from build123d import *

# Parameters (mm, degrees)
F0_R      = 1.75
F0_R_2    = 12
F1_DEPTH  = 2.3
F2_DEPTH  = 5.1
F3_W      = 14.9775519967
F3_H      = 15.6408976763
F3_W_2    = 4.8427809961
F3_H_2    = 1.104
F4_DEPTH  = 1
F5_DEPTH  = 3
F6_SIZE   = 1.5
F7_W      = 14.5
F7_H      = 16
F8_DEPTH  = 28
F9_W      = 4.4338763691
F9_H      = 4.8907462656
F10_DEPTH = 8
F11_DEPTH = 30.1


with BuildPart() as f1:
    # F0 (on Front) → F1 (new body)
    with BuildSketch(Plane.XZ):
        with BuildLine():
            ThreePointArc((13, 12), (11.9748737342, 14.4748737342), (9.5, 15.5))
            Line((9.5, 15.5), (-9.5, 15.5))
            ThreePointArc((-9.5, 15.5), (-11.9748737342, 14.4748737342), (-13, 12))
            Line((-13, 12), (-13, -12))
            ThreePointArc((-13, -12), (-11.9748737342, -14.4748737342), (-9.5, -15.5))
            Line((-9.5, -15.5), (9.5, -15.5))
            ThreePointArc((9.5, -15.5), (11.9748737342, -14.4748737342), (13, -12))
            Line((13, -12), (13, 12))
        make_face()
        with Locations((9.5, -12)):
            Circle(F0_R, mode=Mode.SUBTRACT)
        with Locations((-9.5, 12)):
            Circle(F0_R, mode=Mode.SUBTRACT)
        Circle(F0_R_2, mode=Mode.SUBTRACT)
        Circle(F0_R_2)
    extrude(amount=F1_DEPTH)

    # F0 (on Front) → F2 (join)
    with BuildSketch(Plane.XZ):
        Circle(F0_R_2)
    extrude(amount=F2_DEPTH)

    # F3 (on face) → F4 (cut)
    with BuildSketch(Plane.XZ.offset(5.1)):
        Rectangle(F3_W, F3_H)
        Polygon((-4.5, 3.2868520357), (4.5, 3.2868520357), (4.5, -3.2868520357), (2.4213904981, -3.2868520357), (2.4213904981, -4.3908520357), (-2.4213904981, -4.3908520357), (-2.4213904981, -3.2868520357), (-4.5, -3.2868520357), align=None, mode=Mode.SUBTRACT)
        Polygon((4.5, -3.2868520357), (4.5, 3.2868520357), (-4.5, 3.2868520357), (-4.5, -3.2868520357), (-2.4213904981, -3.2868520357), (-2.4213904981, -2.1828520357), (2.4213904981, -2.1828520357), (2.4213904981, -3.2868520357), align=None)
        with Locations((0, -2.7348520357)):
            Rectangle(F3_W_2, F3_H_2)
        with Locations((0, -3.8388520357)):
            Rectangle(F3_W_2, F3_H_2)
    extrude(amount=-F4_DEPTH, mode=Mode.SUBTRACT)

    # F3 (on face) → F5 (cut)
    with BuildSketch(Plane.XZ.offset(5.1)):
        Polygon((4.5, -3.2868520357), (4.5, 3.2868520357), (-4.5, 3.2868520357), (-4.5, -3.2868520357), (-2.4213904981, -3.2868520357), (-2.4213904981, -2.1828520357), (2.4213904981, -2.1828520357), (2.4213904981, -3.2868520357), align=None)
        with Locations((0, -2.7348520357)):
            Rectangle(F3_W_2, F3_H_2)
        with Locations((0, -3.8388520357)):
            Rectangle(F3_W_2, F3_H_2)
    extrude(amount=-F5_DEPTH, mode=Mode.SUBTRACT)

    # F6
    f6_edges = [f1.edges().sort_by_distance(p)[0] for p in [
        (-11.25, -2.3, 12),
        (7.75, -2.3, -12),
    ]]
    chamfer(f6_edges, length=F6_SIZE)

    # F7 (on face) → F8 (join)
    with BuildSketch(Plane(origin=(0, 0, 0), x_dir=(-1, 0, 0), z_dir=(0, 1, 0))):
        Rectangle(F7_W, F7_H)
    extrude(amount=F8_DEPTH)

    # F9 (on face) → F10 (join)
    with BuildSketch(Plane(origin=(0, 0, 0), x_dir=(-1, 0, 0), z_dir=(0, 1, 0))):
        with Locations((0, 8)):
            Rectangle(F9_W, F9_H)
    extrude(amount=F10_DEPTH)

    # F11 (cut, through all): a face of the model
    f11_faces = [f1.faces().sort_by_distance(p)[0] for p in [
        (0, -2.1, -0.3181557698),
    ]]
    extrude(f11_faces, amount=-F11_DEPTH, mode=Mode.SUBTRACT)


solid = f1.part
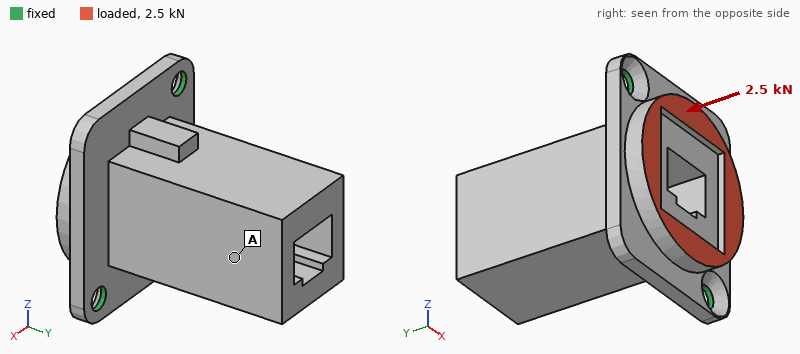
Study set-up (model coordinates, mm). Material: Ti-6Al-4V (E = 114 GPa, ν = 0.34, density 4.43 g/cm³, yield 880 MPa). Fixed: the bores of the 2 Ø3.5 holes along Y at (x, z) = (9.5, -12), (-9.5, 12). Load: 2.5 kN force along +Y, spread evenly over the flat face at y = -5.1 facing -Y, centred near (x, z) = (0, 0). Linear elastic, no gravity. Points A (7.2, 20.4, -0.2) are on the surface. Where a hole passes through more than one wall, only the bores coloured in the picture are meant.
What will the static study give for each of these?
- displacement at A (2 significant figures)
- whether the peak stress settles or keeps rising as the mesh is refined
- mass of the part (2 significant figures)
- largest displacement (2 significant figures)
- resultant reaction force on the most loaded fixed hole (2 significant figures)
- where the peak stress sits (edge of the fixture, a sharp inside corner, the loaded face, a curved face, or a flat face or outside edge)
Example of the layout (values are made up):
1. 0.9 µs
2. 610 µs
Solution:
1. 27 µm
2. keeps rising
3. 32 g
4. 40 µm
5. 1.4 kN
6. edge of the fixture
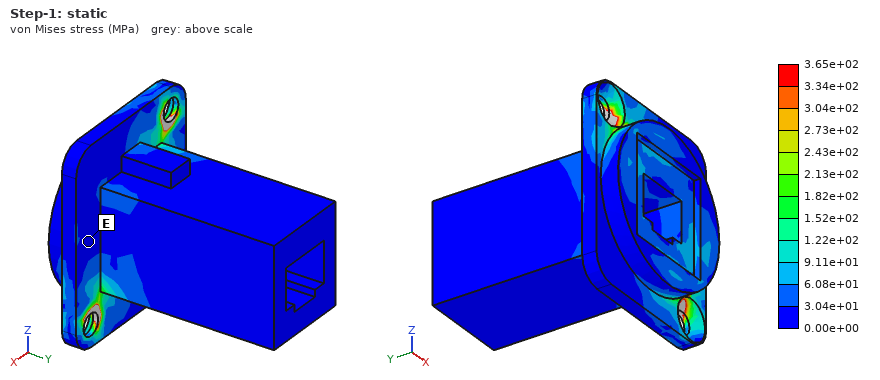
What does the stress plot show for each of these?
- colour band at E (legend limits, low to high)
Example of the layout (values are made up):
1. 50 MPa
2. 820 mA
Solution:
1. 0.00e+00 to 3.04e+01 MPa
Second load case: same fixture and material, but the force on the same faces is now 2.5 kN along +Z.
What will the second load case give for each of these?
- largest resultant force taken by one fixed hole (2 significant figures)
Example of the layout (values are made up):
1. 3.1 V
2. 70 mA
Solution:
1. 1.3 kN
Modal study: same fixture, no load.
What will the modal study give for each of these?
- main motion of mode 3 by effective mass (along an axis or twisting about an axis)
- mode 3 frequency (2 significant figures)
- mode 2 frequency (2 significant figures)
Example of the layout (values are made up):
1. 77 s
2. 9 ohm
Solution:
1. along Y
2. 8200 Hz
3. 6300 Hz
